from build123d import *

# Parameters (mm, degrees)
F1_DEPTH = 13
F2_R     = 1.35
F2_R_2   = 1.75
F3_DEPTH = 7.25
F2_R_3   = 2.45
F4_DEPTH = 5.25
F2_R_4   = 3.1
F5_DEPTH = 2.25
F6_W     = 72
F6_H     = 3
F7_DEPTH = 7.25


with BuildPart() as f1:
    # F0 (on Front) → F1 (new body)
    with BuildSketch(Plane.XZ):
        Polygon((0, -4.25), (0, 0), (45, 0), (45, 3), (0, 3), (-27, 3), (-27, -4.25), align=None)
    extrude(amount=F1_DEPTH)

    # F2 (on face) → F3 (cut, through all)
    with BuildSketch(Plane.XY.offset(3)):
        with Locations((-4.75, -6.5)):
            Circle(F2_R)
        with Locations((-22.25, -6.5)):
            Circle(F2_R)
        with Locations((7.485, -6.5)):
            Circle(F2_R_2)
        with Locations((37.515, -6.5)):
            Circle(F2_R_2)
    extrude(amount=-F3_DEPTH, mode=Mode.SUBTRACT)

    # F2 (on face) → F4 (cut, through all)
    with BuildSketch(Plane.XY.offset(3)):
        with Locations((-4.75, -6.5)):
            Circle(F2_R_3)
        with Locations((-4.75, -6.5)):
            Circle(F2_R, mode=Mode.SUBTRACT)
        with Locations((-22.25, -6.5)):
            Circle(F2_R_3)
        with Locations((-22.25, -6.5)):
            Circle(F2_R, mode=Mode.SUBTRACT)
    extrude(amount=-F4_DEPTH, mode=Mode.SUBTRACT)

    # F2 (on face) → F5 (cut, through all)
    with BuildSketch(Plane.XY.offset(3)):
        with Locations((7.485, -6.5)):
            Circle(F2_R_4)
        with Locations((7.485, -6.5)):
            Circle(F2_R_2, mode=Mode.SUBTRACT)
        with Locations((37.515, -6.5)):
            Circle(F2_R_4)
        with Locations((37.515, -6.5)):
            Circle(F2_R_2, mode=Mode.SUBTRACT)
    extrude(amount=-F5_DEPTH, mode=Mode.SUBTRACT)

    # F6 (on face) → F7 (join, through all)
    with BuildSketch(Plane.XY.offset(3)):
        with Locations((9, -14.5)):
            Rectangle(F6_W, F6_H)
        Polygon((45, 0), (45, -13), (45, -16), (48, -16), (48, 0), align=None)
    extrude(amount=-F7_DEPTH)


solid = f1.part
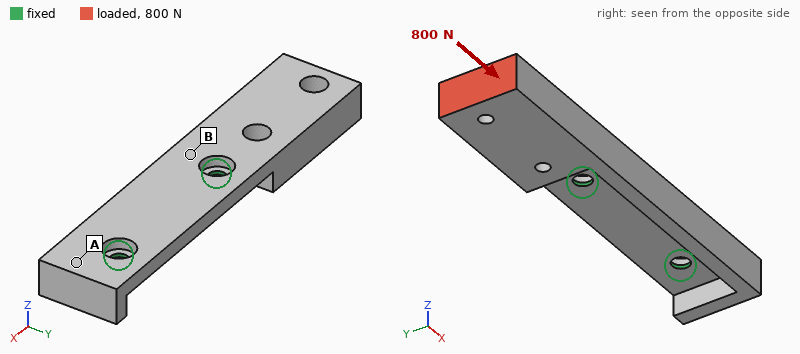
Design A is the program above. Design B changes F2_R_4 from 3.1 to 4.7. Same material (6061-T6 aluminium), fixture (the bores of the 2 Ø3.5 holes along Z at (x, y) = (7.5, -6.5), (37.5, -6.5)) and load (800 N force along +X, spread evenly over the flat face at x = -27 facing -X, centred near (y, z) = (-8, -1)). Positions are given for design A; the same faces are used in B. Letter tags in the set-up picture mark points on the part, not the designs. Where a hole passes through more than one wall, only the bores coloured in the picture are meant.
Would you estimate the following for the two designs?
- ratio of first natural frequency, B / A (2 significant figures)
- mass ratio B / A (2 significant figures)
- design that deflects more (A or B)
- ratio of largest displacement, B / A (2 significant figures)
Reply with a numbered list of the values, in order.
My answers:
1. 0.88
2. 0.97
3. B
4. 1.1
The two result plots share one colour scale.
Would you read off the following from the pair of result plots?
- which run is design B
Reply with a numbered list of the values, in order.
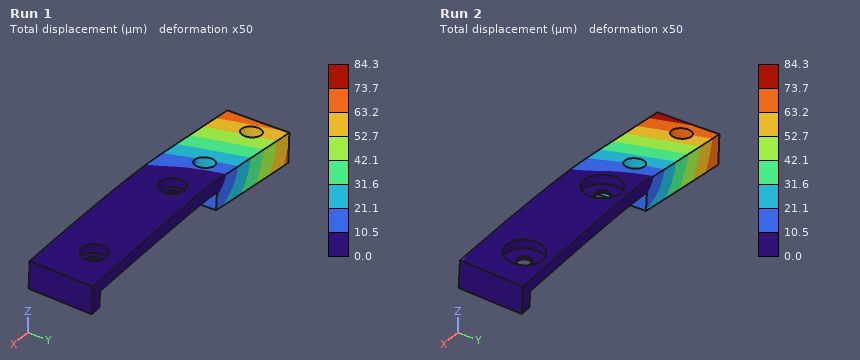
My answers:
1. Run 2
